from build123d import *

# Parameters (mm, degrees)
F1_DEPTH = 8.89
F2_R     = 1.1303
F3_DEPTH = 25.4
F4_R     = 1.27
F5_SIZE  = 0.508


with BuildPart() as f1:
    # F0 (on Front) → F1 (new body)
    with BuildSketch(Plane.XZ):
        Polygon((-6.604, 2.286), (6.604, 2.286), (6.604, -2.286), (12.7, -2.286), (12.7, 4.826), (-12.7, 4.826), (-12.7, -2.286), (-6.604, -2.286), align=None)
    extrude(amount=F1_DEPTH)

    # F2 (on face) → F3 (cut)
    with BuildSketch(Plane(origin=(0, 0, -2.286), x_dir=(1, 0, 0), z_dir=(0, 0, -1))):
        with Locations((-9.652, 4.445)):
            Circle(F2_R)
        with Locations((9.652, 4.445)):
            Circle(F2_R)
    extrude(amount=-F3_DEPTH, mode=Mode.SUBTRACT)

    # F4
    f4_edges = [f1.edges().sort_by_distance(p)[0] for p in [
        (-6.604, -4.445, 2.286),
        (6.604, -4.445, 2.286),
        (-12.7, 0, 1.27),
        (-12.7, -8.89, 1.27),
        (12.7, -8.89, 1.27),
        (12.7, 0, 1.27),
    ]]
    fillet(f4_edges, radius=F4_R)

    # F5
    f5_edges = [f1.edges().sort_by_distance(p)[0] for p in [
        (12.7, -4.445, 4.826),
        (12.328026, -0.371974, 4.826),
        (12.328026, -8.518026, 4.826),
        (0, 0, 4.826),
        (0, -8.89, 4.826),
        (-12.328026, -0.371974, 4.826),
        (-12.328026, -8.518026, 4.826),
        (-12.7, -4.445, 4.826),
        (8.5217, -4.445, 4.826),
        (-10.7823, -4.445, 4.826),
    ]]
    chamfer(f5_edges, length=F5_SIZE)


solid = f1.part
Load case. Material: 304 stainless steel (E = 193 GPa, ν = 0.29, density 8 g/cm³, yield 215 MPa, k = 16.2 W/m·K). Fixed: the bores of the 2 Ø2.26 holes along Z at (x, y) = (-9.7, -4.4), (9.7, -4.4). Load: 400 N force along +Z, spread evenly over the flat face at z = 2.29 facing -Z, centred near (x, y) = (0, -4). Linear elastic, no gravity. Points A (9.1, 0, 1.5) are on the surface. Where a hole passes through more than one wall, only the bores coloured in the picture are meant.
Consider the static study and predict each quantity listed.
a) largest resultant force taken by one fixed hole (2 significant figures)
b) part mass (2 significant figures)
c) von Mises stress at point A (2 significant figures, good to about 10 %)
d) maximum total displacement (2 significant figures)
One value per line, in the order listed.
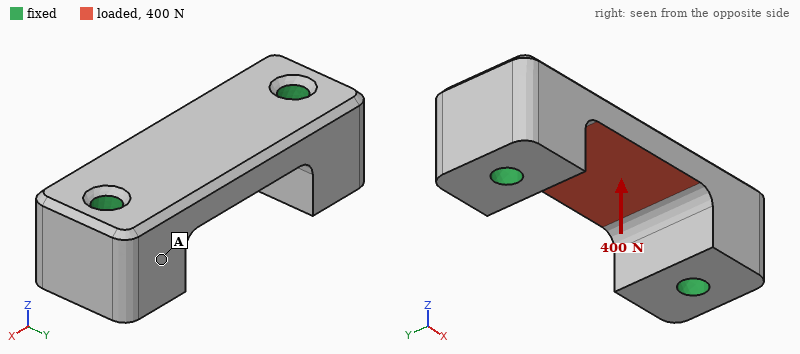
220 N
8.0 g
8.1 MPa
2.9 µm
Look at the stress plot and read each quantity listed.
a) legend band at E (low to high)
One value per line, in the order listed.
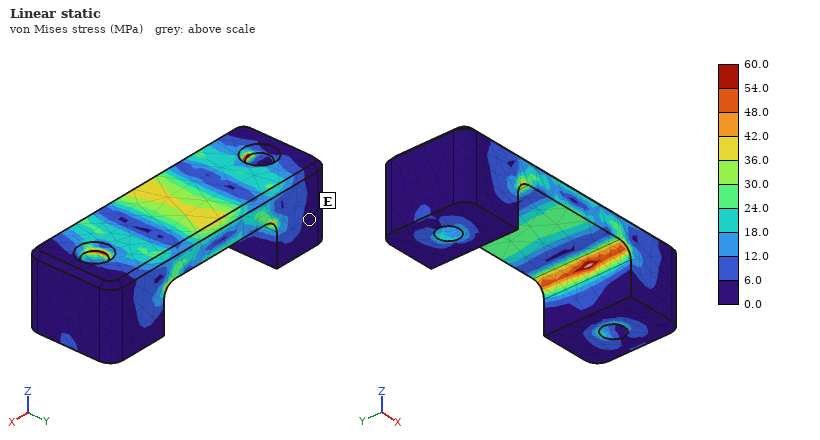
0.0 to 6.0 MPa
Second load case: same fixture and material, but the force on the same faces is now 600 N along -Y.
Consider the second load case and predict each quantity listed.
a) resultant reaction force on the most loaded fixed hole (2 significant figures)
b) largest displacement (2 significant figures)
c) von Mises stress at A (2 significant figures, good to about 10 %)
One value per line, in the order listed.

300 N
3.2 µm
9.2 MPa
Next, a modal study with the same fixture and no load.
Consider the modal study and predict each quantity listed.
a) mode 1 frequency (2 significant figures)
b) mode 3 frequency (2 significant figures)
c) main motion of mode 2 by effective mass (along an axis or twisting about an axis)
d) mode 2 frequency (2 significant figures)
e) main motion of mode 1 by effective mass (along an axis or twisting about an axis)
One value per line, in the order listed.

48 kHz
65 kHz
along Y
58 kHz
along Z
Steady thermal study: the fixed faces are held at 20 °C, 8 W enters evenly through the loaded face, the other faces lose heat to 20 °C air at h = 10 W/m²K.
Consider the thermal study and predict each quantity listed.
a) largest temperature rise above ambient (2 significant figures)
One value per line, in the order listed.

68 K
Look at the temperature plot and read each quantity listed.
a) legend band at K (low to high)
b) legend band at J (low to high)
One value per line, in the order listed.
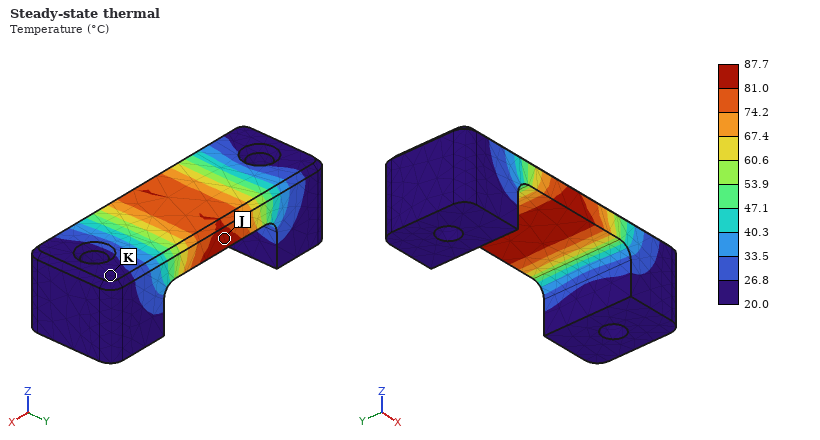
20.0 to 26.8 °C
81.0 to 87.7 °C
